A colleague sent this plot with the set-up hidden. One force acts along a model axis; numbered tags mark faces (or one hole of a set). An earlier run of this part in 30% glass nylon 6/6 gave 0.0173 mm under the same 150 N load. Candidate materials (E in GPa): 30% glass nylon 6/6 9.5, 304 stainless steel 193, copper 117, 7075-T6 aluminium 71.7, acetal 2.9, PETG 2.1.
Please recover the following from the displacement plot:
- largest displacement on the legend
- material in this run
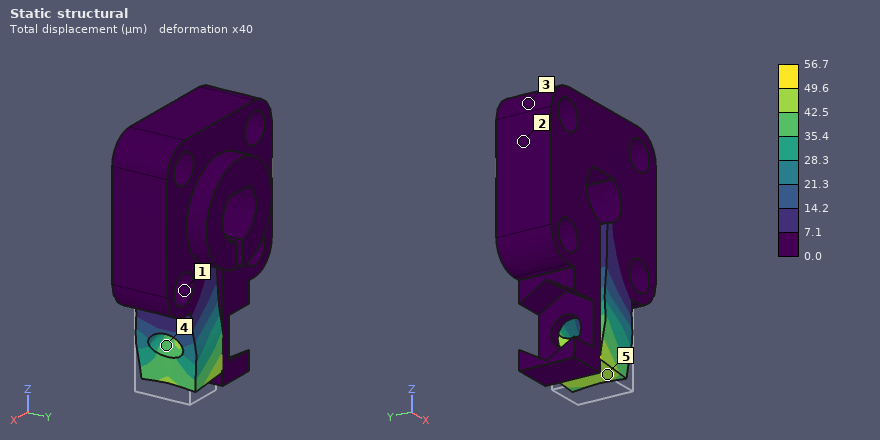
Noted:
56.7 µm
acetal
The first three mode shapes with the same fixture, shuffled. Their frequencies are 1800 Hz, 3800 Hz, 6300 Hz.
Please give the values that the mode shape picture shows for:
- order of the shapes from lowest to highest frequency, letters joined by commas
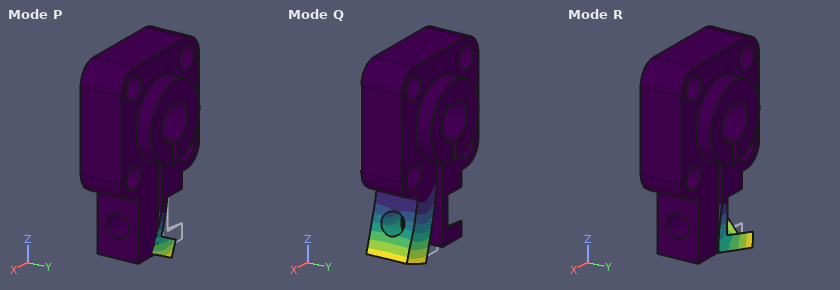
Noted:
P, R, Q
